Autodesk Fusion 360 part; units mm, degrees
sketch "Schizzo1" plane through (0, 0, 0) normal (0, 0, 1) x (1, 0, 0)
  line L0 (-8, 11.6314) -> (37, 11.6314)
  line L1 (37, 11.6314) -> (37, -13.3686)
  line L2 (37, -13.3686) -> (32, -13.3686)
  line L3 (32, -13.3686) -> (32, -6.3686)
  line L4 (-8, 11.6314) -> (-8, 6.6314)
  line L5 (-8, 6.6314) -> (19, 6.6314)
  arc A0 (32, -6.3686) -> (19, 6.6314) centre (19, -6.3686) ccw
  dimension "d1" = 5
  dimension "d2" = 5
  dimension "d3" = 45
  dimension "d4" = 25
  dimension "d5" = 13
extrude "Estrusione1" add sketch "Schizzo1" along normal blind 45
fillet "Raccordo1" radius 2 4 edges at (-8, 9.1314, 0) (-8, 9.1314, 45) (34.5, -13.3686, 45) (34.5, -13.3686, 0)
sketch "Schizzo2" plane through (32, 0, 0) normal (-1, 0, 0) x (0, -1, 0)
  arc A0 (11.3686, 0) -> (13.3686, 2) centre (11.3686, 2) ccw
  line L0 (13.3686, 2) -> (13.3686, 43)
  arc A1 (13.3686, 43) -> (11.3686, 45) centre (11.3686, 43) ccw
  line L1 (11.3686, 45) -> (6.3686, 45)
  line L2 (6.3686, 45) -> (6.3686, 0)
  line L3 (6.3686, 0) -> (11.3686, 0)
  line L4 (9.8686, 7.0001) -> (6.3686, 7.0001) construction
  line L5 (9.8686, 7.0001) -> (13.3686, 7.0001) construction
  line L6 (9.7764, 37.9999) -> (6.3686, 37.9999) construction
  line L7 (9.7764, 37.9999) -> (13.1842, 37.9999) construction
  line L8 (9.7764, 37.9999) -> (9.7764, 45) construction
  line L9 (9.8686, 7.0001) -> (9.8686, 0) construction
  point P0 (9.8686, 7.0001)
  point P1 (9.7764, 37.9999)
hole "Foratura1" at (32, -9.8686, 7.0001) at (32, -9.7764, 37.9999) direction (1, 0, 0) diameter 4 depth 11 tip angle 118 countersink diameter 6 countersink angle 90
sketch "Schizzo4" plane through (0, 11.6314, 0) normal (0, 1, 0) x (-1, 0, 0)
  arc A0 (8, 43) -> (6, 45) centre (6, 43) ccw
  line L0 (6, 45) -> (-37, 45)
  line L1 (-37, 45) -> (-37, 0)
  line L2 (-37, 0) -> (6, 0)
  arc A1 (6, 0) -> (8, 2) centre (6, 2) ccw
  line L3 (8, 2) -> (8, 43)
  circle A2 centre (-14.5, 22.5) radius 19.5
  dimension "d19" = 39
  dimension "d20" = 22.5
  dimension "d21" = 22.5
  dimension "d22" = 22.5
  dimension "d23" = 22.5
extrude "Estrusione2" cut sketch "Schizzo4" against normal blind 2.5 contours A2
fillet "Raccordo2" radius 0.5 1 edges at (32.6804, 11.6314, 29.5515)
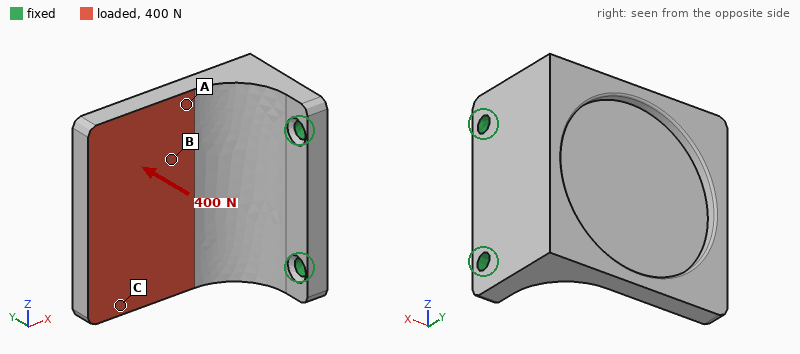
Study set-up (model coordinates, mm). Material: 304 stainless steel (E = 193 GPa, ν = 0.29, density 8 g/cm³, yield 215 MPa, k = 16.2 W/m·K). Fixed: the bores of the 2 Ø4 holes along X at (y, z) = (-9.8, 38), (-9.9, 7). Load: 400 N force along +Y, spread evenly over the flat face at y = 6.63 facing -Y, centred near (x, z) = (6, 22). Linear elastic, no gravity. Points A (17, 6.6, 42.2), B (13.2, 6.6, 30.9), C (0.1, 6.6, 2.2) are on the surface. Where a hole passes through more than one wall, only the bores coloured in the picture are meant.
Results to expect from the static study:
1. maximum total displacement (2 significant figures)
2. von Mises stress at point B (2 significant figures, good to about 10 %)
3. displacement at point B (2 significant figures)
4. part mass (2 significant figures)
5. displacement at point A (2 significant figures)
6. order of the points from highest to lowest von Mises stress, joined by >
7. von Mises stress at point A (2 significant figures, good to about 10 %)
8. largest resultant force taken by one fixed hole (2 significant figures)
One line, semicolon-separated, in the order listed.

0.16 mm; 29 MPa; 0.056 mm; 100 g; 0.042 mm; A > B > C; 55 MPa; 220 N
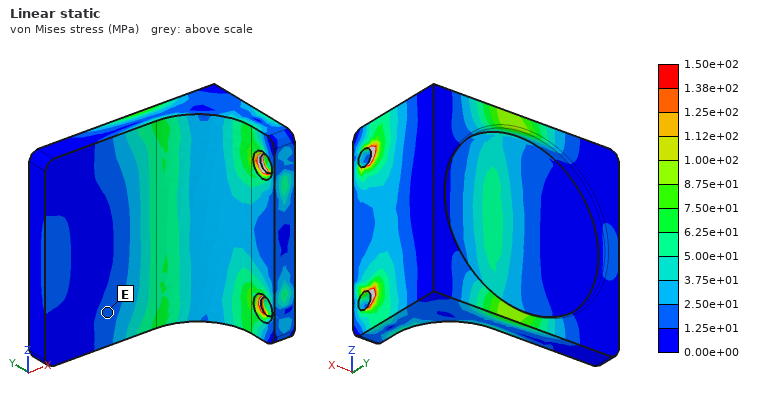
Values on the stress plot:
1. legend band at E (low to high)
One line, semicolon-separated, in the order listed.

1.25e+01 to 2.50e+01 MPa
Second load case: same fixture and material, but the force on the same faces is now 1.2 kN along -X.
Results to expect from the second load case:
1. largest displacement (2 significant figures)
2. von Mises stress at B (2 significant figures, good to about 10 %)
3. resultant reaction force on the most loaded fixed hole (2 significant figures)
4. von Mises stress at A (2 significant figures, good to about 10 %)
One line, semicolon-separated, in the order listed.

75 µm; 21 MPa; 600 N; 30 MPa
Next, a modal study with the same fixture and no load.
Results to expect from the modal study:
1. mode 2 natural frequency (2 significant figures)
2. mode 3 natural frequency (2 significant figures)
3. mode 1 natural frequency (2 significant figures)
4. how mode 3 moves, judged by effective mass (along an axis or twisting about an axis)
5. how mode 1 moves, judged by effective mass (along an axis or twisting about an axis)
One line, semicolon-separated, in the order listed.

3600 Hz; 4500 Hz; 1500 Hz; along X; along Y
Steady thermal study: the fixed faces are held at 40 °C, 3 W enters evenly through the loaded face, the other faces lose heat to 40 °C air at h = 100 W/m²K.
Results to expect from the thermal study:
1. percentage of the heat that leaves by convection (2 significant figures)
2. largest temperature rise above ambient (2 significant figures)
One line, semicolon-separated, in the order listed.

87 %; 12 K
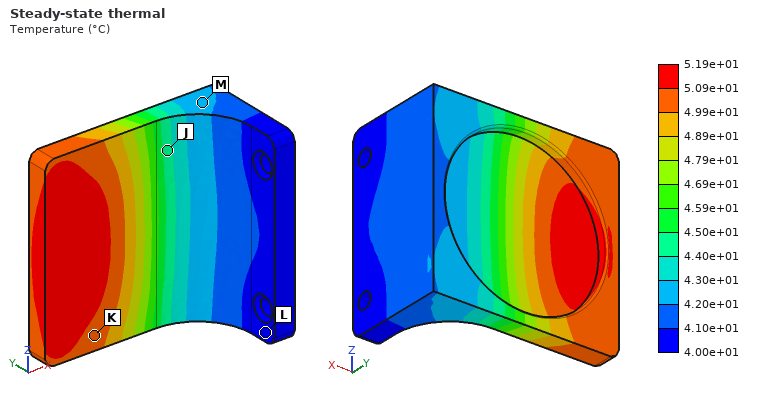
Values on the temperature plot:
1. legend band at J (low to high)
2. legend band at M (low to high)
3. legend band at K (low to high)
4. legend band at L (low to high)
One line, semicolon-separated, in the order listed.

4.40e+01 to 4.50e+01 °C; 4.20e+01 to 4.30e+01 °C; 4.99e+01 to 5.09e+01 °C; 4.00e+01 to 4.10e+01 °C
